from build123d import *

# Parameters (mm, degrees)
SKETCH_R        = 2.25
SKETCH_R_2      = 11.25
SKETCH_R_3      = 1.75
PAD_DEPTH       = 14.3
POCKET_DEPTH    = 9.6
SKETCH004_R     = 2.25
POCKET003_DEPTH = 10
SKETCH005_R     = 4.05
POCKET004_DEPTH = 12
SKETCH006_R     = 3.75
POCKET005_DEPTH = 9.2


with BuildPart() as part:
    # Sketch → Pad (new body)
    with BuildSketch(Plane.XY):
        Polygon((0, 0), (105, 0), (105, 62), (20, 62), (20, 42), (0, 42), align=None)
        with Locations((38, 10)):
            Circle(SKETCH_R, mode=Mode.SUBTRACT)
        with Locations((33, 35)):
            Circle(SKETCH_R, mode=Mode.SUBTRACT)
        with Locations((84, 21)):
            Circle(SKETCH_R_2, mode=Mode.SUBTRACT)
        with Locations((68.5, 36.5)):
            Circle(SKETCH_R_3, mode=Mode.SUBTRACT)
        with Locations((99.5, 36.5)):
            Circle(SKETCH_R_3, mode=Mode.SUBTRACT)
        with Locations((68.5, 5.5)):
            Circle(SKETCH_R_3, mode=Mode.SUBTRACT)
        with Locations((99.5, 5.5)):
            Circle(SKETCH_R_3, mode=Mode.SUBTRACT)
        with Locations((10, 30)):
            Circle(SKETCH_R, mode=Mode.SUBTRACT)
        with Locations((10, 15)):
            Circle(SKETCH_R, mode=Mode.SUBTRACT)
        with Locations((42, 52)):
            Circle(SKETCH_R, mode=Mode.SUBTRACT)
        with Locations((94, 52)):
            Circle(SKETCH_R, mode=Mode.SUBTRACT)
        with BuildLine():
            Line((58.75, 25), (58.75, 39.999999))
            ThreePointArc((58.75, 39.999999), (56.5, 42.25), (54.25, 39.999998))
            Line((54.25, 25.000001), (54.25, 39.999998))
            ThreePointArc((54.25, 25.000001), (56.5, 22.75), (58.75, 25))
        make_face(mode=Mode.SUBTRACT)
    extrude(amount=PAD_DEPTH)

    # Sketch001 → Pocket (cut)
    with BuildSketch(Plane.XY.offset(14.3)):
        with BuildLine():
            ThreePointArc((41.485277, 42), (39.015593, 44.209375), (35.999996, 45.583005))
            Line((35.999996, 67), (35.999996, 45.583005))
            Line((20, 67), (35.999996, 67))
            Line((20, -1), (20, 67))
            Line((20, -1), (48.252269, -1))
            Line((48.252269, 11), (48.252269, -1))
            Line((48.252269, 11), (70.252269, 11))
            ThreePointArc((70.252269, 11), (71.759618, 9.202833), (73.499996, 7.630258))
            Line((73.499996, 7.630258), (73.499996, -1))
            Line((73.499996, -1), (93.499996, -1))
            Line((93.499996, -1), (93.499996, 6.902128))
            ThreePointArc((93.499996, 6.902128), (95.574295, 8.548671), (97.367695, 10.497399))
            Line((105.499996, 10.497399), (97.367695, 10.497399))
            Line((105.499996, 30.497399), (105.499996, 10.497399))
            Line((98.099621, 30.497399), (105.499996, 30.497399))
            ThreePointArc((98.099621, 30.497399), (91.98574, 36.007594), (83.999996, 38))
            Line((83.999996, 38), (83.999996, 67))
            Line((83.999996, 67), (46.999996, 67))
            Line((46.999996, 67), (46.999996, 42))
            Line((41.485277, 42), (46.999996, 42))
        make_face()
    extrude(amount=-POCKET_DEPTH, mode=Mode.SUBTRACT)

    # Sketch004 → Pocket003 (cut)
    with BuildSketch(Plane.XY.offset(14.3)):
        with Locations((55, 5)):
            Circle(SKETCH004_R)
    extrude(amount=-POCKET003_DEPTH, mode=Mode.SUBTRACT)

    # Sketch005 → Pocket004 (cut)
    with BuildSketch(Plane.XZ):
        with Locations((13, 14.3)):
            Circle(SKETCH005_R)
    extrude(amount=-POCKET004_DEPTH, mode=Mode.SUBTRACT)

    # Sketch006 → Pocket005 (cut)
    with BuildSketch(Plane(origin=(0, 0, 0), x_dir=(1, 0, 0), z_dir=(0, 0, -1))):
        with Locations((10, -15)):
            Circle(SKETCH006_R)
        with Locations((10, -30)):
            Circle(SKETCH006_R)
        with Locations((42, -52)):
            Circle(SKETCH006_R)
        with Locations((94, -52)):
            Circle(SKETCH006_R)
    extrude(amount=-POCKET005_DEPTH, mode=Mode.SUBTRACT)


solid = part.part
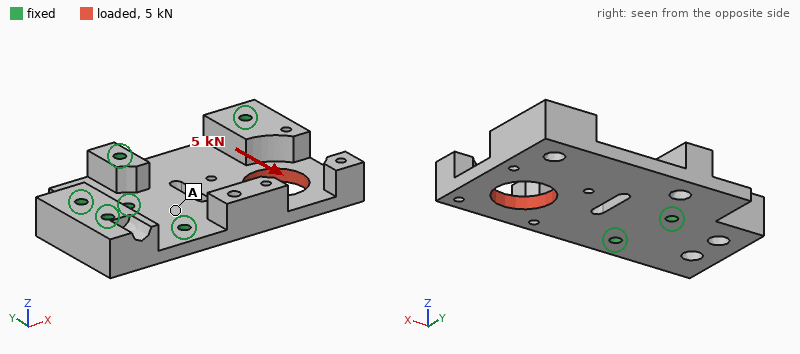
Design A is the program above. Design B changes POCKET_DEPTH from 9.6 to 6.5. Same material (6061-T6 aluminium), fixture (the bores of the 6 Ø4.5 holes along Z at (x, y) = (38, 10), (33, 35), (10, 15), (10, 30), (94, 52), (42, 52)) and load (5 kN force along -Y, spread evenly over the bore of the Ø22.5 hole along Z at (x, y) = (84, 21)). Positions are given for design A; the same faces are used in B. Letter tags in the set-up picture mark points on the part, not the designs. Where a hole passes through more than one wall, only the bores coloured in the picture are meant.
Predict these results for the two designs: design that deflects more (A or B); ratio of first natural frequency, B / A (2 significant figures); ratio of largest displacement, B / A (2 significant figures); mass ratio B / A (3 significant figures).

A
1.4
0.59
1.26
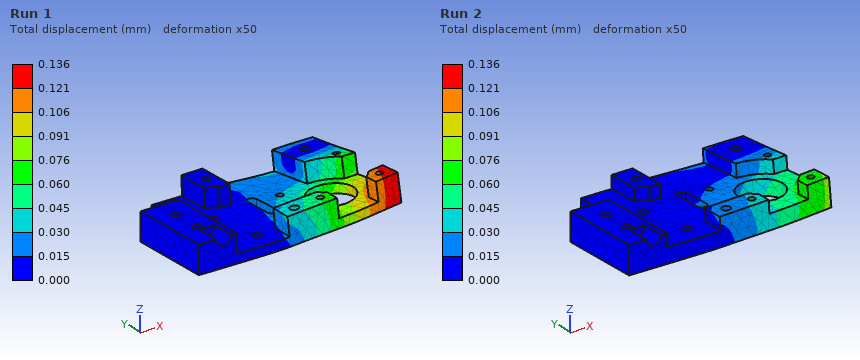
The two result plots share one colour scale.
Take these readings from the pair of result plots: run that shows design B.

Run 2
